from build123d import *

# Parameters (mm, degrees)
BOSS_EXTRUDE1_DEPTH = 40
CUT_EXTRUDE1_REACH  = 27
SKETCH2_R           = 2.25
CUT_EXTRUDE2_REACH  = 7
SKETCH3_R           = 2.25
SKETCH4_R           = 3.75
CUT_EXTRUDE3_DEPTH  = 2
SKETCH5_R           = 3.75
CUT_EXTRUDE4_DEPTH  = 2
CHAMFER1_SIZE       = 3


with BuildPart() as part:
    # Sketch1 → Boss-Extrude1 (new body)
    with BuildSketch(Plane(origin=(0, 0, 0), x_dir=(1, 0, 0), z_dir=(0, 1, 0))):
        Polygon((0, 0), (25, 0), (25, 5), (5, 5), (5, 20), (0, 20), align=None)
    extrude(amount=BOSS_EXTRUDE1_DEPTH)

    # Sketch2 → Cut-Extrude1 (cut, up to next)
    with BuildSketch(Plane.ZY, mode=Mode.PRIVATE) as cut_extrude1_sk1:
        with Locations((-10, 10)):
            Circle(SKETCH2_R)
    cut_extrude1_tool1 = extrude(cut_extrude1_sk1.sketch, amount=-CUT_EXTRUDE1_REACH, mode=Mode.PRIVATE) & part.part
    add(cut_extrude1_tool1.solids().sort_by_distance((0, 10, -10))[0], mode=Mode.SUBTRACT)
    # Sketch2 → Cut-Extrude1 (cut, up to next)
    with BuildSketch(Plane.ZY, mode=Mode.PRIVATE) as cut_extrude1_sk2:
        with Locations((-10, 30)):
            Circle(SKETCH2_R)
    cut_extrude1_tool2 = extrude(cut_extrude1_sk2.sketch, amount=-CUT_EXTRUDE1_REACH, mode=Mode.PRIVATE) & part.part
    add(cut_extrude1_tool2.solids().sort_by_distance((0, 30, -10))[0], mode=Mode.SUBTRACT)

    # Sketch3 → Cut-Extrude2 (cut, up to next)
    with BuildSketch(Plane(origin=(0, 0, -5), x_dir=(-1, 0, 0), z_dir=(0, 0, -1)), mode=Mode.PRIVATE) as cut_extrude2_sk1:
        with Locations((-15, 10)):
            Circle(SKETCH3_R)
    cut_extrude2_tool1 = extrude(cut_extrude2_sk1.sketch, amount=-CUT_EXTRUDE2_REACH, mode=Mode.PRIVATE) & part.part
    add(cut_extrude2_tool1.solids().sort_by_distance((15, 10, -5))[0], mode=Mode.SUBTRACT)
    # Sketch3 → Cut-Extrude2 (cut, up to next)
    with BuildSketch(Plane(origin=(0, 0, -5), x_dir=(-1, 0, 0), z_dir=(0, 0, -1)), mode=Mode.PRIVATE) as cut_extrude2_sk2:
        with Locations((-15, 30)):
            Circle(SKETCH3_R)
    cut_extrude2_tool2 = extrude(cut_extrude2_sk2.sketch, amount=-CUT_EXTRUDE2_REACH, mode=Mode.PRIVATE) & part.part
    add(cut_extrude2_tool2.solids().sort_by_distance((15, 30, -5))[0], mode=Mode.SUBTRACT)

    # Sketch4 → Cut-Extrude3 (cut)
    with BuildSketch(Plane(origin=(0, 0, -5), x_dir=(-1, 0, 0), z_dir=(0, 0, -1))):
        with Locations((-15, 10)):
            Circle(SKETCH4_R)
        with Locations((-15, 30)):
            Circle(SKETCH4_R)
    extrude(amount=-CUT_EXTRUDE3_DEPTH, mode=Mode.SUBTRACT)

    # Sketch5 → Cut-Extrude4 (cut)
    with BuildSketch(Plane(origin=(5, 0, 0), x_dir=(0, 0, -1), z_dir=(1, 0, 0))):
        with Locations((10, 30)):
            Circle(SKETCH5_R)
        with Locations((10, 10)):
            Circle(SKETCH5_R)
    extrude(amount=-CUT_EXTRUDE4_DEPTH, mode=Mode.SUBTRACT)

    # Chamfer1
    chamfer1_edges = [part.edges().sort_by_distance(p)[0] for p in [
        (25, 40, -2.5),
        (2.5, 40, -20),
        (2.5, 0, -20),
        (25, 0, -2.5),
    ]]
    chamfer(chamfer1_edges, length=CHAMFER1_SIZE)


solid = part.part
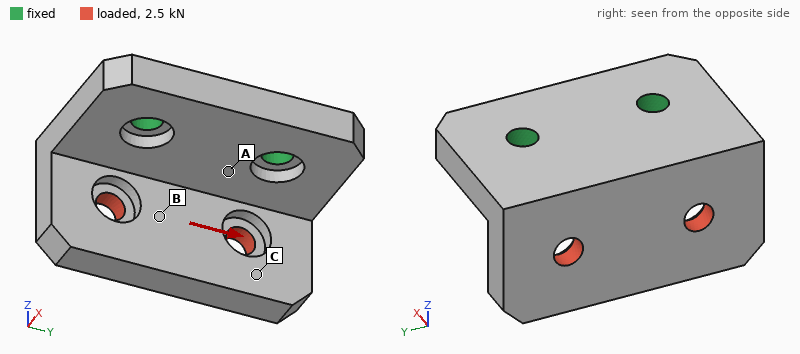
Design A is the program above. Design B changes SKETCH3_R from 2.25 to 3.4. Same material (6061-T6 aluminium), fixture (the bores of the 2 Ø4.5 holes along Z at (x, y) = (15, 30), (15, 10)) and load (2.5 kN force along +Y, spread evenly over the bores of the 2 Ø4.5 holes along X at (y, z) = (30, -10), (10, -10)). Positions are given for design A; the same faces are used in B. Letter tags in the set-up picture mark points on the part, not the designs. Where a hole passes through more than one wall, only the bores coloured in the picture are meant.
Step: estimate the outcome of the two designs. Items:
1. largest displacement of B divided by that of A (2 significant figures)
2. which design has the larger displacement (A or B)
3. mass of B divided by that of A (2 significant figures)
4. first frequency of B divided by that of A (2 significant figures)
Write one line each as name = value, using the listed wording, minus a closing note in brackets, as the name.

largest displacement of B divided by that of A = 0.76
which design has the larger displacement = A
mass of B divided by that of A = 0.98
first frequency of B divided by that of A = 1.2
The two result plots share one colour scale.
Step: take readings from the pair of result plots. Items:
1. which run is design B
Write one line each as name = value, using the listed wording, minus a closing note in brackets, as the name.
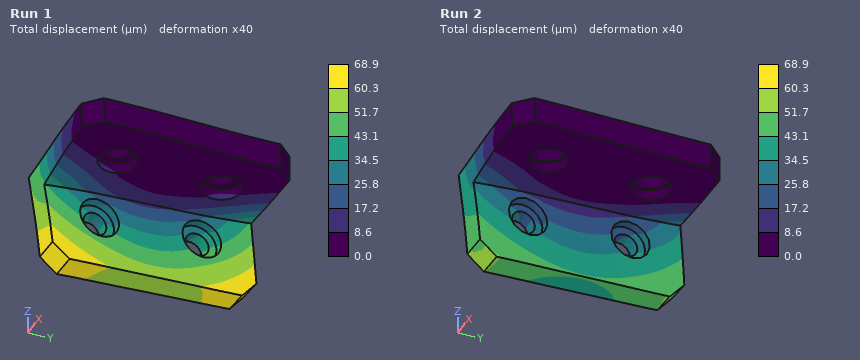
which run is design B = Run 2
